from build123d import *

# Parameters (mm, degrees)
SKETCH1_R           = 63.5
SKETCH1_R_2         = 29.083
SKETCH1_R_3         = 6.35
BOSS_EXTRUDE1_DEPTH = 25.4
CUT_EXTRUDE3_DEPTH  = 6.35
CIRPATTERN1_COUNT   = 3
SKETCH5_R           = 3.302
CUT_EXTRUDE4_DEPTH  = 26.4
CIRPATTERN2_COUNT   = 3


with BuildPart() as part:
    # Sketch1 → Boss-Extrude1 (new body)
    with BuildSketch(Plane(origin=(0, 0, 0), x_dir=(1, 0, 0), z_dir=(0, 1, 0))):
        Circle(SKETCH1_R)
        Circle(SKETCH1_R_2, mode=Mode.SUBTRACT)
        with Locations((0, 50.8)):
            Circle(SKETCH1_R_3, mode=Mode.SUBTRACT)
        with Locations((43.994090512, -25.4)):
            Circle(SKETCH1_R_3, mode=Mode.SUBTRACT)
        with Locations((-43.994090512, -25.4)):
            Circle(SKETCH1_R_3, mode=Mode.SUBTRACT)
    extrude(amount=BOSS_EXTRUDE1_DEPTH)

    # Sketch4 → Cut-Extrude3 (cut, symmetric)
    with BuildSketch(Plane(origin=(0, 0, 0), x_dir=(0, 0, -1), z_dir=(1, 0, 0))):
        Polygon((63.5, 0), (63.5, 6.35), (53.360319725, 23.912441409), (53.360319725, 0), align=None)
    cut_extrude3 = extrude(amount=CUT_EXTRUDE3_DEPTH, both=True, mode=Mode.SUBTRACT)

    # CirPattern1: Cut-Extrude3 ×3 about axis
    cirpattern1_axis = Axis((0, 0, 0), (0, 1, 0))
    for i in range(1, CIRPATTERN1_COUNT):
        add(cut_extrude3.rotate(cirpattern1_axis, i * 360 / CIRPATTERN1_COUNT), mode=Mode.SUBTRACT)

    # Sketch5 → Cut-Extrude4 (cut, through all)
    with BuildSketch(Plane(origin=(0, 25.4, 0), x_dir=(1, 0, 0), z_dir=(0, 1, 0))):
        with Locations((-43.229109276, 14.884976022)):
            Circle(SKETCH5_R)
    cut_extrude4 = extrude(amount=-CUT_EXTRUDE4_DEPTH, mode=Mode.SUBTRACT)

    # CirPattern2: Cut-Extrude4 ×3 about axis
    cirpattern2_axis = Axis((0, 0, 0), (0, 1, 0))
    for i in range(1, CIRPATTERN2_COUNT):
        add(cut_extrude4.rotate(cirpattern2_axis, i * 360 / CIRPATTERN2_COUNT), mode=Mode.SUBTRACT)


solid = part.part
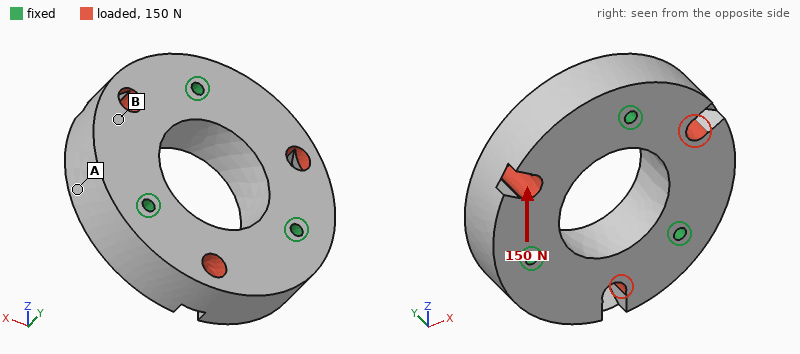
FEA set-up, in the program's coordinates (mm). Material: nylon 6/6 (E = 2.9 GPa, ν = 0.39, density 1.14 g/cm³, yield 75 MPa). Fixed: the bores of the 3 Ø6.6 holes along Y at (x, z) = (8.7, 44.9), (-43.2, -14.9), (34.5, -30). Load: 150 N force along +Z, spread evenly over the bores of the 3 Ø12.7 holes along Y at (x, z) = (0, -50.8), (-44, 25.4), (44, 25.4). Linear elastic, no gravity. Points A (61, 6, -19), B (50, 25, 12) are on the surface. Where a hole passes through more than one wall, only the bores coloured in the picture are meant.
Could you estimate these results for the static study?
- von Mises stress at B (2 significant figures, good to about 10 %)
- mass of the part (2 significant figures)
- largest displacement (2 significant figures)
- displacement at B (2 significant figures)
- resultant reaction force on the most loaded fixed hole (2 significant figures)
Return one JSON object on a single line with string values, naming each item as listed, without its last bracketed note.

{"von Mises stress at B": "0.069 MPa", "mass of the part": "270 g", "largest displacement": "2.3 µm", "displacement at B": "0.91 µm", "resultant reaction force on the most loaded fixed hole": "68 N"}
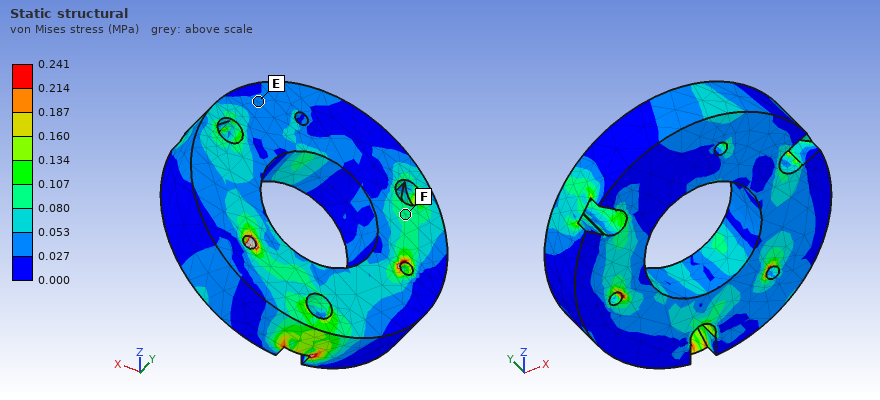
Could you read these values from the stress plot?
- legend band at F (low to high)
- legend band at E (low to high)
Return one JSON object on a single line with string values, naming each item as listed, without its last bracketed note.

{"legend band at F": "0.080 to 0.107 MPa", "legend band at E": "0.027 to 0.053 MPa"}
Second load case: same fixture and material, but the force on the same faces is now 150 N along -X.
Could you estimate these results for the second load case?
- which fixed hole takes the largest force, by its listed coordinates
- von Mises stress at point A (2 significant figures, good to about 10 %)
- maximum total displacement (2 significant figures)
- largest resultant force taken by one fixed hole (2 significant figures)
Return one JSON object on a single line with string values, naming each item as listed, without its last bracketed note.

{"which fixed hole takes the largest force, by its listed coordinates": "(8.7, 44.9)", "von Mises stress at point A": "0.025 MPa", "maximum total displacement": "2.1 µm", "largest resultant force taken by one fixed hole": "75 N"}
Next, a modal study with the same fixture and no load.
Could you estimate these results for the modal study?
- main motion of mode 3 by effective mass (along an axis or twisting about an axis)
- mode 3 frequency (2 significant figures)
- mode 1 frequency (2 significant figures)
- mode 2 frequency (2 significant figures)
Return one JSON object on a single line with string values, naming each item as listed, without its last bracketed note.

{"main motion of mode 3 by effective mass": "along Y", "mode 3 frequency": "2800 Hz", "mode 1 frequency": "2400 Hz", "mode 2 frequency": "2400 Hz"}
